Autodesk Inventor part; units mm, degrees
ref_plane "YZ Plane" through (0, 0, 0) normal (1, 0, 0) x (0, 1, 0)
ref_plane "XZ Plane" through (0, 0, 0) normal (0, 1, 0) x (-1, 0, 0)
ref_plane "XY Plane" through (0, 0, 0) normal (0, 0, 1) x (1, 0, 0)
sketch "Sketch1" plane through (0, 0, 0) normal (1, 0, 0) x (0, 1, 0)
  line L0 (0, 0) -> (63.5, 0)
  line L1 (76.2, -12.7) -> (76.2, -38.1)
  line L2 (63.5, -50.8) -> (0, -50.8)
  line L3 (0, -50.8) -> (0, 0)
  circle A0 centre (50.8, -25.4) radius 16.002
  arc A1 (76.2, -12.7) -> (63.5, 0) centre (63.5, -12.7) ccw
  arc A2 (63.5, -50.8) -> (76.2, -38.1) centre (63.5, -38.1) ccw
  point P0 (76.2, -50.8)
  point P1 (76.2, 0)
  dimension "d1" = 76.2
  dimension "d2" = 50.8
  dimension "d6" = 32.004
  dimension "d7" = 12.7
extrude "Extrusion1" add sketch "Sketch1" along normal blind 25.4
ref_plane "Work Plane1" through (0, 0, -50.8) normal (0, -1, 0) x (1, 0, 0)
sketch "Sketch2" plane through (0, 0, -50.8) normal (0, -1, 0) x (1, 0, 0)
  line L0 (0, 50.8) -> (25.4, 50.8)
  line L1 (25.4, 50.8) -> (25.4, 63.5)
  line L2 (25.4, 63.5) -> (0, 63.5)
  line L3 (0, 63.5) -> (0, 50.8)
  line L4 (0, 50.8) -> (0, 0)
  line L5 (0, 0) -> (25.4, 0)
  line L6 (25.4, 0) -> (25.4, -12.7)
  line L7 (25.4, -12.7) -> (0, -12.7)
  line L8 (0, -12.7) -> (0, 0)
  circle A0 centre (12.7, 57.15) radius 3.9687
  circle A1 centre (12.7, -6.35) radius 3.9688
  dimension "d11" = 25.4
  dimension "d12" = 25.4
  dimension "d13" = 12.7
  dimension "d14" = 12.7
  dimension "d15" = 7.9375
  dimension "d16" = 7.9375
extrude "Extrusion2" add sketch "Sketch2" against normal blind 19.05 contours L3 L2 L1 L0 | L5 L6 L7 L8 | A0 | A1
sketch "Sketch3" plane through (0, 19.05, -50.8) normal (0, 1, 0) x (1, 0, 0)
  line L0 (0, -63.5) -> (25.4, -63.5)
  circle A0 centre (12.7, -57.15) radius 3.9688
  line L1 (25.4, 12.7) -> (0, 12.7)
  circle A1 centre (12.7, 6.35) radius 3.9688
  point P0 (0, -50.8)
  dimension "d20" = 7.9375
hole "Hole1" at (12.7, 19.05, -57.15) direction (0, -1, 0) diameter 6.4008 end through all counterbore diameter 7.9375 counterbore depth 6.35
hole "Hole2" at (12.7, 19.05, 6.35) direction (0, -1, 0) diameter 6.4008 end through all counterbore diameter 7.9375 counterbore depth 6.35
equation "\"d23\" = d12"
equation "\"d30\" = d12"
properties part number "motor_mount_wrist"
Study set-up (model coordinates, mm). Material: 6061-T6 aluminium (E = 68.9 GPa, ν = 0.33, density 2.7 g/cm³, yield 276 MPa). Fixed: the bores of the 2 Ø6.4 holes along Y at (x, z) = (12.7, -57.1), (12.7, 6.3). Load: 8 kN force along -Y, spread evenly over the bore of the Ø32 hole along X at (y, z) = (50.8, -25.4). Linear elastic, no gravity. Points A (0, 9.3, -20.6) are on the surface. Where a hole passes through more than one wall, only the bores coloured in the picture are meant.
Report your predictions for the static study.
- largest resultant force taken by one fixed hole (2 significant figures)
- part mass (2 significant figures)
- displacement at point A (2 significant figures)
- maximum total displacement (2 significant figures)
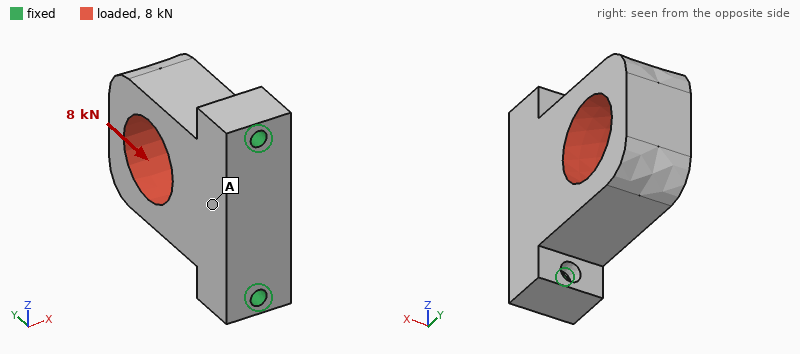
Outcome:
4.3 kN
230 g
8.2 µm
19 µm
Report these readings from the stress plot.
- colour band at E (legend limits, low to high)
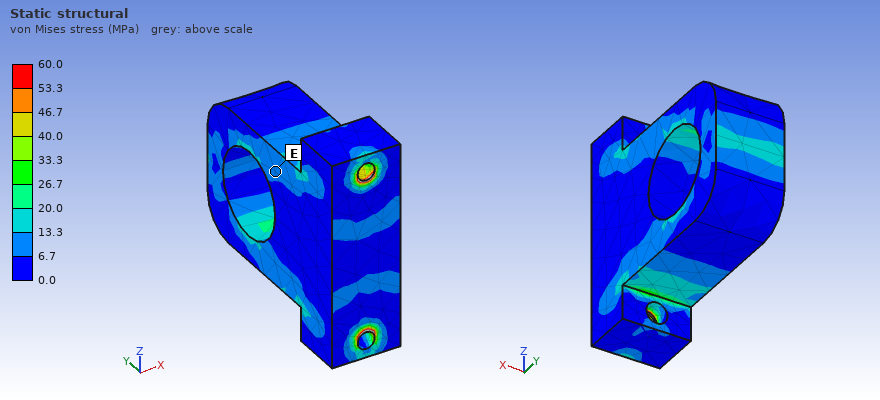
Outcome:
6.7 to 13.3 MPa
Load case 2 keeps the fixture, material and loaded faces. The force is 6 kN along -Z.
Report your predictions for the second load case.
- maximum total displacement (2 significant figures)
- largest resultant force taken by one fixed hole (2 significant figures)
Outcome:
60 µm
5.3 kN
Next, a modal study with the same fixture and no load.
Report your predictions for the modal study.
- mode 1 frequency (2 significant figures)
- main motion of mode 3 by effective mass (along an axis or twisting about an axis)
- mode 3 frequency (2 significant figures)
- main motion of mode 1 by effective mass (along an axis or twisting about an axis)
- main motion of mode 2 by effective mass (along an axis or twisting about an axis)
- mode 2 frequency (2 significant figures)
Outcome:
2400 Hz
twisting about Y
7500 Hz
along X
along Z
5300 Hz
